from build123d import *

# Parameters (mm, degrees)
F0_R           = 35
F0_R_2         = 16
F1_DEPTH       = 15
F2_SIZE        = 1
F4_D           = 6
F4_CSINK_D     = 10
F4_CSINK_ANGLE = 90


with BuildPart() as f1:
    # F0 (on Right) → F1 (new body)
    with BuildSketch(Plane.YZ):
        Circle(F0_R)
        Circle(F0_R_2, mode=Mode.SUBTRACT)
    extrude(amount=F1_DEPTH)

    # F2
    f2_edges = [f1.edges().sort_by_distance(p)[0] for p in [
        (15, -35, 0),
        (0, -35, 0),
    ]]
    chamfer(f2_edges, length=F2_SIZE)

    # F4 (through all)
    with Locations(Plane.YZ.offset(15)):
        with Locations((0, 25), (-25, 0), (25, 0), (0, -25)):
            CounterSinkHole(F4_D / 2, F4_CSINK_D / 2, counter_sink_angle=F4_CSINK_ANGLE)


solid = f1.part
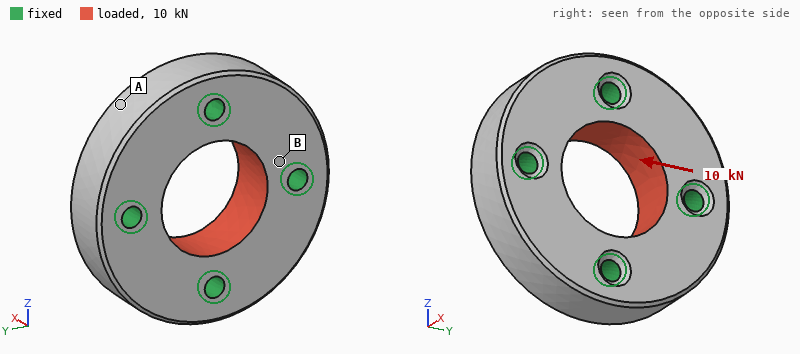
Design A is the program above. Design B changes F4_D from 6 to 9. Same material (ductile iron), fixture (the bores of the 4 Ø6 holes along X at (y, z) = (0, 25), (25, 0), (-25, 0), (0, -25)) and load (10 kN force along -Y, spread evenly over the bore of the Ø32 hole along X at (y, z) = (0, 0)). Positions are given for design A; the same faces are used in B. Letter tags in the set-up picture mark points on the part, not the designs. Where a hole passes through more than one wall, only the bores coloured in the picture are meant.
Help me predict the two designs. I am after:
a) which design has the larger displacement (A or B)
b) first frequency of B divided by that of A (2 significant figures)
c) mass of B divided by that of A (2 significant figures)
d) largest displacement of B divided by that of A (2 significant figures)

A
1.3
0.96
0.78
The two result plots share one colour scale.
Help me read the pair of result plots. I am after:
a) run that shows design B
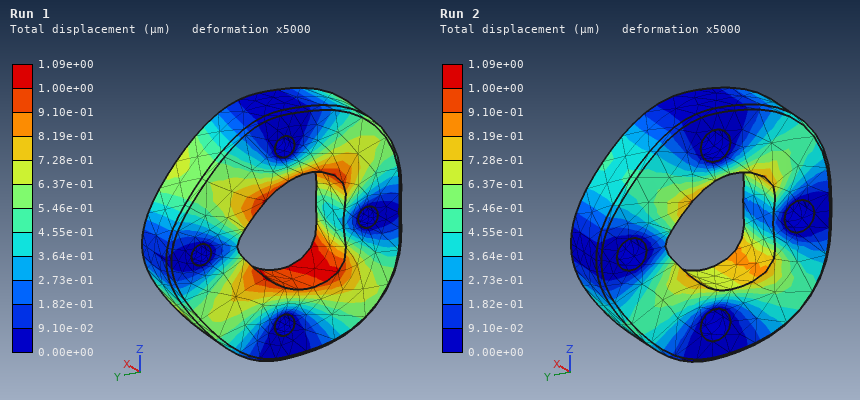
Run 2
